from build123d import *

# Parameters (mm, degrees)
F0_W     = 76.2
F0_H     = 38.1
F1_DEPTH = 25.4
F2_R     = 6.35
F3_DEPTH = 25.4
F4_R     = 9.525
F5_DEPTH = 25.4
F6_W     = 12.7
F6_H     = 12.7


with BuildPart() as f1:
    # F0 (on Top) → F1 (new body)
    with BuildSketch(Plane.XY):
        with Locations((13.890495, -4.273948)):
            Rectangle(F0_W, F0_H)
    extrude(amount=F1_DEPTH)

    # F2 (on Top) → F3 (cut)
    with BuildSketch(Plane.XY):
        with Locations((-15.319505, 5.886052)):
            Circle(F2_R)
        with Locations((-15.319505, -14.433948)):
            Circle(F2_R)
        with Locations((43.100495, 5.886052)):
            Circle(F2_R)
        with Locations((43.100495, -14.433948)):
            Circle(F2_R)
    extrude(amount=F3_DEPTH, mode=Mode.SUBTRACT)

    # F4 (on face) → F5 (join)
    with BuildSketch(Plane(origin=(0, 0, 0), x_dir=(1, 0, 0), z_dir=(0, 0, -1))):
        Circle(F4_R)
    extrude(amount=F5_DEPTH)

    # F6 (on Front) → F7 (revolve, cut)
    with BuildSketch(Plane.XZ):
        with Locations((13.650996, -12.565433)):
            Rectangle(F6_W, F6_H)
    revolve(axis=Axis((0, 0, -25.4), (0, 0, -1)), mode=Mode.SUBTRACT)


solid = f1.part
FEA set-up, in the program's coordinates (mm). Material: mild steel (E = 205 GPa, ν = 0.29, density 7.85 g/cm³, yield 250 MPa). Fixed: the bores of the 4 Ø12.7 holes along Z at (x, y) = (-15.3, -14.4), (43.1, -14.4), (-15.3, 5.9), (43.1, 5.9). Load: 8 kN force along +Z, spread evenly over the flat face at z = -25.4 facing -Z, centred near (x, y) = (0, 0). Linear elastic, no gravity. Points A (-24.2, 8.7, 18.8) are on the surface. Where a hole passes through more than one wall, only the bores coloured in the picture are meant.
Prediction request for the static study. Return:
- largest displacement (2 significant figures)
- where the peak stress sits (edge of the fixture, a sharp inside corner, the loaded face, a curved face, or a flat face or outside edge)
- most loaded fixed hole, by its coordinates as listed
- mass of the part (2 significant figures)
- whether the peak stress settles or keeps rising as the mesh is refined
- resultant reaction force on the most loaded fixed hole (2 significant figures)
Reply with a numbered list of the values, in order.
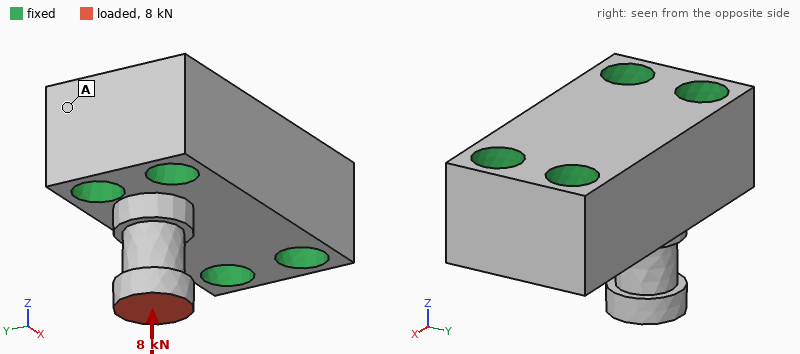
1. 7.8 µm
2. edge of the fixture
3. (-15.3, 5.9)
4. 520 g
5. keeps rising
6. 4.3 kN
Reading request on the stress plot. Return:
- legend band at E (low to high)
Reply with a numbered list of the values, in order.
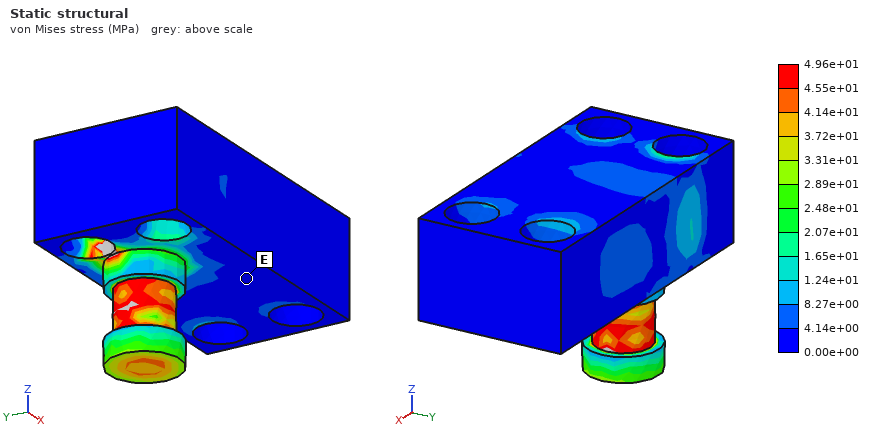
1. 0.00e+00 to 4.14e+00 MPa
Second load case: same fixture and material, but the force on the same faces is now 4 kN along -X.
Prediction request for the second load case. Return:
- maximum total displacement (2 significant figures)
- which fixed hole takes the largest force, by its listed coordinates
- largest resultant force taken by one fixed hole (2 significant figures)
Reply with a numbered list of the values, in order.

1. 55 µm
2. (-15.3, 5.9)
3. 3.3 kN
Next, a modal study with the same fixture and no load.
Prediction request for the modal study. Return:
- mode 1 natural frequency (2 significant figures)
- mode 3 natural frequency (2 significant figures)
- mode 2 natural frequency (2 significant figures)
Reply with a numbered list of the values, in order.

1. 12 kHz
2. 24 kHz
3. 12 kHz
